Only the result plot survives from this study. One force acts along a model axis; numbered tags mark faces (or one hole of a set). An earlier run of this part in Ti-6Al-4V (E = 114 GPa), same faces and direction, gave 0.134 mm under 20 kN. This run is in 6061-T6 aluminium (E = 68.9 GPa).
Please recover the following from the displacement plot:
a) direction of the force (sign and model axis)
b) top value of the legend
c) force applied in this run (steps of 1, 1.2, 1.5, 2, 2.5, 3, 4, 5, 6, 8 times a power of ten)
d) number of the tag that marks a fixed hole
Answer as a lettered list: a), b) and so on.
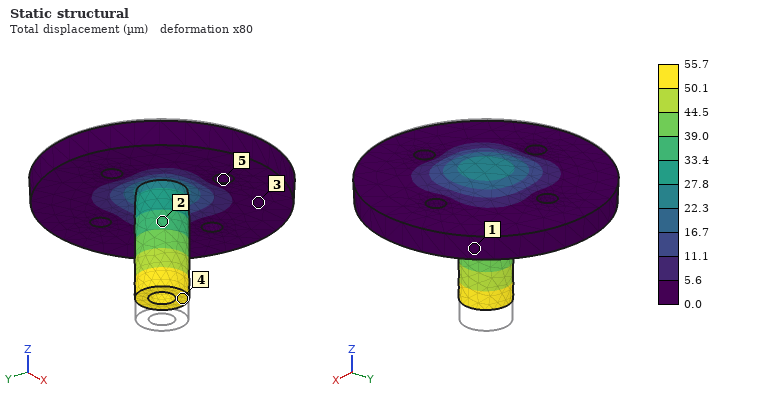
a) +Z
b) 55.7 µm
c) 5 kN
d) 5
